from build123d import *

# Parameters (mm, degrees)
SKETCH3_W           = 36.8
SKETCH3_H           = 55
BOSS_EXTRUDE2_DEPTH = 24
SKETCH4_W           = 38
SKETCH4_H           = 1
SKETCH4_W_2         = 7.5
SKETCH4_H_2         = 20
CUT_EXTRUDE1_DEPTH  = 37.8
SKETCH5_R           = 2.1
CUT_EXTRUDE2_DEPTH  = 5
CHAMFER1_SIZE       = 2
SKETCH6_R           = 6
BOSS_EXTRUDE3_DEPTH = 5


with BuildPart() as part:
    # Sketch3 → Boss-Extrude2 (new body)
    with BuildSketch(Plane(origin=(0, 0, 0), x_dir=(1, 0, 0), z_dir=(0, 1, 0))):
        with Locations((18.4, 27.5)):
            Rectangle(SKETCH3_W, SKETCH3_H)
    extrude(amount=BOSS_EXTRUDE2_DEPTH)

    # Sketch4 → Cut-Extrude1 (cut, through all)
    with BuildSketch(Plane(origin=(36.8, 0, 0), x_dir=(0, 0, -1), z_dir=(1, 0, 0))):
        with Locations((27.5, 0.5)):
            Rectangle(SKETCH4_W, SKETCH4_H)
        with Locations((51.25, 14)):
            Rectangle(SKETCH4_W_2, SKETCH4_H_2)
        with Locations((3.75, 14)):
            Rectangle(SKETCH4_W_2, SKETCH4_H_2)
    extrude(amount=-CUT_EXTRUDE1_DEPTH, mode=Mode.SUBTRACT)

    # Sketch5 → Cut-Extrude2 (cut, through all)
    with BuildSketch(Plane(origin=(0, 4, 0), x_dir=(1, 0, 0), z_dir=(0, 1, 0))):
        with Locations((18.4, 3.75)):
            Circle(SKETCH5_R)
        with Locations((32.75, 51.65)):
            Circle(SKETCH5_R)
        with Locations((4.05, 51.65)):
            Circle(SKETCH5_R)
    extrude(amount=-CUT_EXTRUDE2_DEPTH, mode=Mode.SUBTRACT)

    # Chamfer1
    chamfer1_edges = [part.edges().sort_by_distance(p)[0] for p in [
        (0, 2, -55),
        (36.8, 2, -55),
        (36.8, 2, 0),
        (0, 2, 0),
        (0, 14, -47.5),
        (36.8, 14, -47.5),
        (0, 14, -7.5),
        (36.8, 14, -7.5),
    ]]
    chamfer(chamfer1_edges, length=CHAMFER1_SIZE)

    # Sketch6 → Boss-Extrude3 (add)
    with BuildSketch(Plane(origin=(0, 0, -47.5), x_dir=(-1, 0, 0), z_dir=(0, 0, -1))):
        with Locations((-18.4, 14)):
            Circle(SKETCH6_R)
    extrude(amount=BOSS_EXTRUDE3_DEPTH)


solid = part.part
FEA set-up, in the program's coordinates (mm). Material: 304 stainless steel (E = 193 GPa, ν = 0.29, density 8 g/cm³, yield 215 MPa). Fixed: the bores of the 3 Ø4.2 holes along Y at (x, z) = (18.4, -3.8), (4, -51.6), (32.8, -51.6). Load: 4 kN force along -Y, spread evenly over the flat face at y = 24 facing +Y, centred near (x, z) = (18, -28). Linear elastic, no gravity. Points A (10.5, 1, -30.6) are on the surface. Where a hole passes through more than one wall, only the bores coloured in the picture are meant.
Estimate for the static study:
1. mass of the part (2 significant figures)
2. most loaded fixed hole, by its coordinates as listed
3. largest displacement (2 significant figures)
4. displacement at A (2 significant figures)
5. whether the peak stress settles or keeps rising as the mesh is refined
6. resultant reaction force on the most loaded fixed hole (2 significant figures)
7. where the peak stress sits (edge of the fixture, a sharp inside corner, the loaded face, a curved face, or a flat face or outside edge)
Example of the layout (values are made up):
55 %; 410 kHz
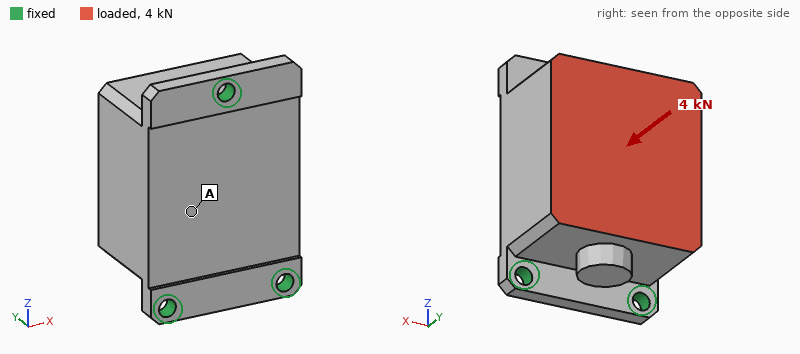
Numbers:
290 g; (18.4, -3.8); 5.3 µm; 4.4 µm; keeps rising; 2.3 kN; edge of the fixture
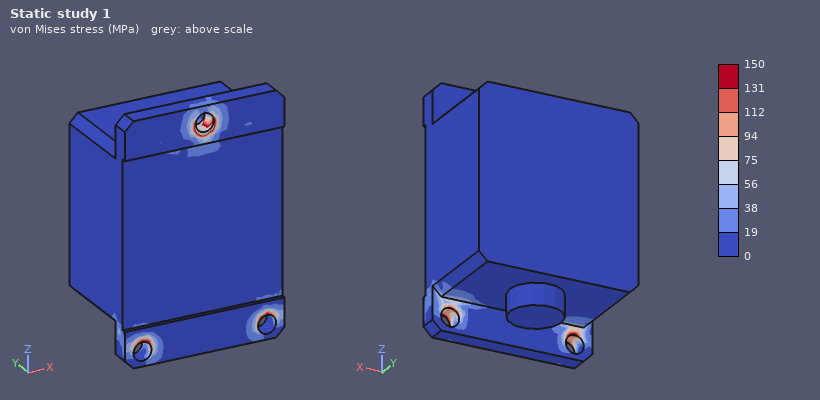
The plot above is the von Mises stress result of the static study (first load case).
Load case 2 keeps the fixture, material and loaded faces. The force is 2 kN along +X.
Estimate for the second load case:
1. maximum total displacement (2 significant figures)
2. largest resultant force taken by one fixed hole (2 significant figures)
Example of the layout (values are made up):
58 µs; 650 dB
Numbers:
13 µm; 1.9 kN
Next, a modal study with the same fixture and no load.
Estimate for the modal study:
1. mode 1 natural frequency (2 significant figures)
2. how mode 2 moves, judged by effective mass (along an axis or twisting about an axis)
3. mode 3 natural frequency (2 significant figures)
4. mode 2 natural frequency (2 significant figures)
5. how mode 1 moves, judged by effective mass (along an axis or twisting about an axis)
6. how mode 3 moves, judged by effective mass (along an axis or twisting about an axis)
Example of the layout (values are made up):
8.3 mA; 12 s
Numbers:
5900 Hz; along Y; 11 kHz; 8900 Hz; along X; along Z
